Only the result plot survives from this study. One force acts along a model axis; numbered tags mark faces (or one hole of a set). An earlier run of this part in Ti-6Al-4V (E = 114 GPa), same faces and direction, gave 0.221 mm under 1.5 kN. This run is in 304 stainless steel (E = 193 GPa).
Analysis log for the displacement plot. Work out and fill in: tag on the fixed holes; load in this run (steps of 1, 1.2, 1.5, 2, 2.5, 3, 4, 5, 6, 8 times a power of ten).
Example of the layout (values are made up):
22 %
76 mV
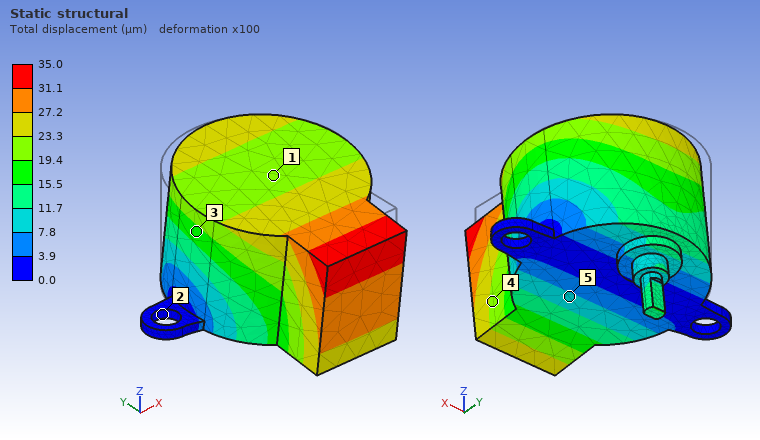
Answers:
2
400 N
